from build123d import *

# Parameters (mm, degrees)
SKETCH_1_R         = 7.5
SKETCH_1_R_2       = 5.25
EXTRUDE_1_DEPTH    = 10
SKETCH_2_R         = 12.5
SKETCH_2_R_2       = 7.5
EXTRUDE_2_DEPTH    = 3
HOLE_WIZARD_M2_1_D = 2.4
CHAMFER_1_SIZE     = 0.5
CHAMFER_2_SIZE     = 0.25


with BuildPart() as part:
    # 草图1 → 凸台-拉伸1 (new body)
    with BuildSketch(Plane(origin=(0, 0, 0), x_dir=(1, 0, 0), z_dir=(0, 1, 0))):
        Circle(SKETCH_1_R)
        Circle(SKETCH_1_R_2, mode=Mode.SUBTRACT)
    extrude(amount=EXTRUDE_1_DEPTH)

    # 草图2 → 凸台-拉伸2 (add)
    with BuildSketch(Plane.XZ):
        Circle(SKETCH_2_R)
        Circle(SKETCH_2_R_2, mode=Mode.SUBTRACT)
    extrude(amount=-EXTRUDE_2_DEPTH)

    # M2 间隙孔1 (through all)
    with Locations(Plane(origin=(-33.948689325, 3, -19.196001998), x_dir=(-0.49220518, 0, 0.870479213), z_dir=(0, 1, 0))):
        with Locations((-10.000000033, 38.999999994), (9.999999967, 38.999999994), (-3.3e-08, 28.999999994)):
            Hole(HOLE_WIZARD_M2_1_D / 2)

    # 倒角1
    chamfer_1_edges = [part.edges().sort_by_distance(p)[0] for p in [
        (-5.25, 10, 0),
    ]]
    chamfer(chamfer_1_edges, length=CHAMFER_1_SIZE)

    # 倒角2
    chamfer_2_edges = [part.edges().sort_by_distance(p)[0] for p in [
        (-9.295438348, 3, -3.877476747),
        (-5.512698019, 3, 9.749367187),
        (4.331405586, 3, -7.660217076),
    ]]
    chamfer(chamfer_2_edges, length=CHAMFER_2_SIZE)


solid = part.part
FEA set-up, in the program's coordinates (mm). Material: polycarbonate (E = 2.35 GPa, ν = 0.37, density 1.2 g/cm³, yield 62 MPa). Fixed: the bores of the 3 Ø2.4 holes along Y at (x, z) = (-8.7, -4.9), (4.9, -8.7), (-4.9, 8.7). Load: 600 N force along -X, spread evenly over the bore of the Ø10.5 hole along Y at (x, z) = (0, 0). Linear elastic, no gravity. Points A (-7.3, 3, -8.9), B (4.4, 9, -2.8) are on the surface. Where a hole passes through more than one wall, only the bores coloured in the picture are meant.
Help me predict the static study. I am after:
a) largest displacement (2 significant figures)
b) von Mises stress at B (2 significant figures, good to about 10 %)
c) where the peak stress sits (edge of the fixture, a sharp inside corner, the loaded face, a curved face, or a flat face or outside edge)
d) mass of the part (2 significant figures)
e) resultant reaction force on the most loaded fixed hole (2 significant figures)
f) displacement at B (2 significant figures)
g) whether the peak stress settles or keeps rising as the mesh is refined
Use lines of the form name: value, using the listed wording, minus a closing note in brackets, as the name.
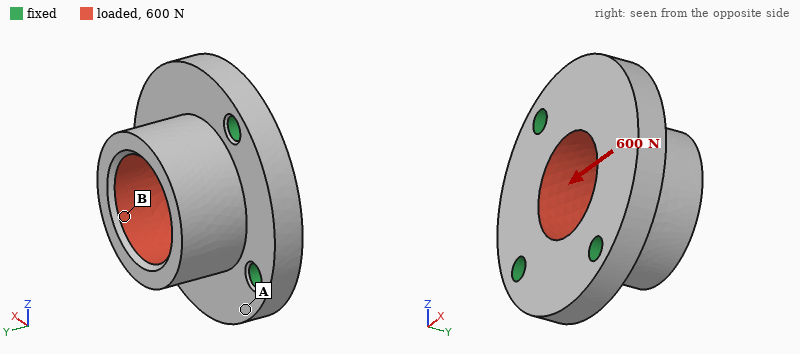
largest displacement: 0.28 mm
von Mises stress at B: 12 MPa
where the peak stress sits: edge of the fixture
mass of the part: 2.2 g
resultant reaction force on the most loaded fixed hole: 240 N
displacement at B: 0.18 mm
whether the peak stress settles or keeps rising as the mesh is refined: keeps rising
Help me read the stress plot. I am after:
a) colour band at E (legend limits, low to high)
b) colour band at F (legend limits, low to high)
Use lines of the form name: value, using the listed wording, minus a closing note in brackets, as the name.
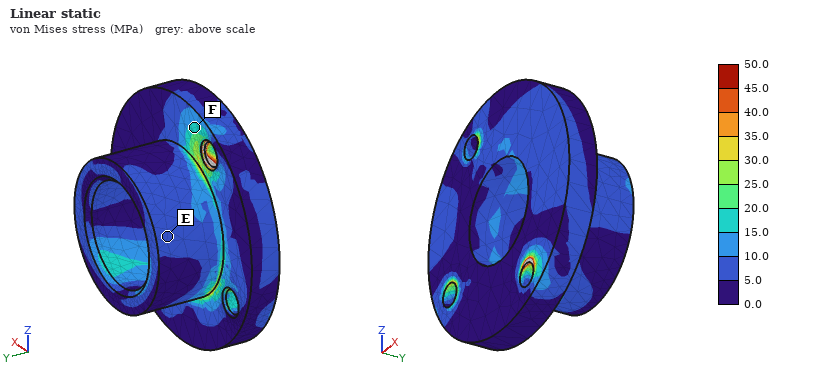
colour band at E: 5.0 to 10.0 MPa
colour band at F: 15.0 to 20.0 MPa
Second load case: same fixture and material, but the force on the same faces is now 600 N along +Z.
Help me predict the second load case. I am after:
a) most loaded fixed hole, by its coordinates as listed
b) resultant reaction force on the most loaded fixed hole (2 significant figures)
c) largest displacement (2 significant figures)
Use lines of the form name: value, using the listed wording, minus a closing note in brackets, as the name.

most loaded fixed hole, by its coordinates as listed: (4.9, -8.7)
resultant reaction force on the most loaded fixed hole: 270 N
largest displacement: 0.18 mm
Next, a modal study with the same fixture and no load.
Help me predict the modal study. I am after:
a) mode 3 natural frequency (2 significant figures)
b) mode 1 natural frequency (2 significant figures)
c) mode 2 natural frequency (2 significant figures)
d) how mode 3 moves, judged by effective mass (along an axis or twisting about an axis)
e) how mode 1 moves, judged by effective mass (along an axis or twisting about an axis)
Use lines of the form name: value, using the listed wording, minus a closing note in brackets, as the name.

mode 3 natural frequency: 12 kHz
mode 1 natural frequency: 4600 Hz
mode 2 natural frequency: 11 kHz
how mode 3 moves, judged by effective mass: along Z
how mode 1 moves, judged by effective mass: along Y
